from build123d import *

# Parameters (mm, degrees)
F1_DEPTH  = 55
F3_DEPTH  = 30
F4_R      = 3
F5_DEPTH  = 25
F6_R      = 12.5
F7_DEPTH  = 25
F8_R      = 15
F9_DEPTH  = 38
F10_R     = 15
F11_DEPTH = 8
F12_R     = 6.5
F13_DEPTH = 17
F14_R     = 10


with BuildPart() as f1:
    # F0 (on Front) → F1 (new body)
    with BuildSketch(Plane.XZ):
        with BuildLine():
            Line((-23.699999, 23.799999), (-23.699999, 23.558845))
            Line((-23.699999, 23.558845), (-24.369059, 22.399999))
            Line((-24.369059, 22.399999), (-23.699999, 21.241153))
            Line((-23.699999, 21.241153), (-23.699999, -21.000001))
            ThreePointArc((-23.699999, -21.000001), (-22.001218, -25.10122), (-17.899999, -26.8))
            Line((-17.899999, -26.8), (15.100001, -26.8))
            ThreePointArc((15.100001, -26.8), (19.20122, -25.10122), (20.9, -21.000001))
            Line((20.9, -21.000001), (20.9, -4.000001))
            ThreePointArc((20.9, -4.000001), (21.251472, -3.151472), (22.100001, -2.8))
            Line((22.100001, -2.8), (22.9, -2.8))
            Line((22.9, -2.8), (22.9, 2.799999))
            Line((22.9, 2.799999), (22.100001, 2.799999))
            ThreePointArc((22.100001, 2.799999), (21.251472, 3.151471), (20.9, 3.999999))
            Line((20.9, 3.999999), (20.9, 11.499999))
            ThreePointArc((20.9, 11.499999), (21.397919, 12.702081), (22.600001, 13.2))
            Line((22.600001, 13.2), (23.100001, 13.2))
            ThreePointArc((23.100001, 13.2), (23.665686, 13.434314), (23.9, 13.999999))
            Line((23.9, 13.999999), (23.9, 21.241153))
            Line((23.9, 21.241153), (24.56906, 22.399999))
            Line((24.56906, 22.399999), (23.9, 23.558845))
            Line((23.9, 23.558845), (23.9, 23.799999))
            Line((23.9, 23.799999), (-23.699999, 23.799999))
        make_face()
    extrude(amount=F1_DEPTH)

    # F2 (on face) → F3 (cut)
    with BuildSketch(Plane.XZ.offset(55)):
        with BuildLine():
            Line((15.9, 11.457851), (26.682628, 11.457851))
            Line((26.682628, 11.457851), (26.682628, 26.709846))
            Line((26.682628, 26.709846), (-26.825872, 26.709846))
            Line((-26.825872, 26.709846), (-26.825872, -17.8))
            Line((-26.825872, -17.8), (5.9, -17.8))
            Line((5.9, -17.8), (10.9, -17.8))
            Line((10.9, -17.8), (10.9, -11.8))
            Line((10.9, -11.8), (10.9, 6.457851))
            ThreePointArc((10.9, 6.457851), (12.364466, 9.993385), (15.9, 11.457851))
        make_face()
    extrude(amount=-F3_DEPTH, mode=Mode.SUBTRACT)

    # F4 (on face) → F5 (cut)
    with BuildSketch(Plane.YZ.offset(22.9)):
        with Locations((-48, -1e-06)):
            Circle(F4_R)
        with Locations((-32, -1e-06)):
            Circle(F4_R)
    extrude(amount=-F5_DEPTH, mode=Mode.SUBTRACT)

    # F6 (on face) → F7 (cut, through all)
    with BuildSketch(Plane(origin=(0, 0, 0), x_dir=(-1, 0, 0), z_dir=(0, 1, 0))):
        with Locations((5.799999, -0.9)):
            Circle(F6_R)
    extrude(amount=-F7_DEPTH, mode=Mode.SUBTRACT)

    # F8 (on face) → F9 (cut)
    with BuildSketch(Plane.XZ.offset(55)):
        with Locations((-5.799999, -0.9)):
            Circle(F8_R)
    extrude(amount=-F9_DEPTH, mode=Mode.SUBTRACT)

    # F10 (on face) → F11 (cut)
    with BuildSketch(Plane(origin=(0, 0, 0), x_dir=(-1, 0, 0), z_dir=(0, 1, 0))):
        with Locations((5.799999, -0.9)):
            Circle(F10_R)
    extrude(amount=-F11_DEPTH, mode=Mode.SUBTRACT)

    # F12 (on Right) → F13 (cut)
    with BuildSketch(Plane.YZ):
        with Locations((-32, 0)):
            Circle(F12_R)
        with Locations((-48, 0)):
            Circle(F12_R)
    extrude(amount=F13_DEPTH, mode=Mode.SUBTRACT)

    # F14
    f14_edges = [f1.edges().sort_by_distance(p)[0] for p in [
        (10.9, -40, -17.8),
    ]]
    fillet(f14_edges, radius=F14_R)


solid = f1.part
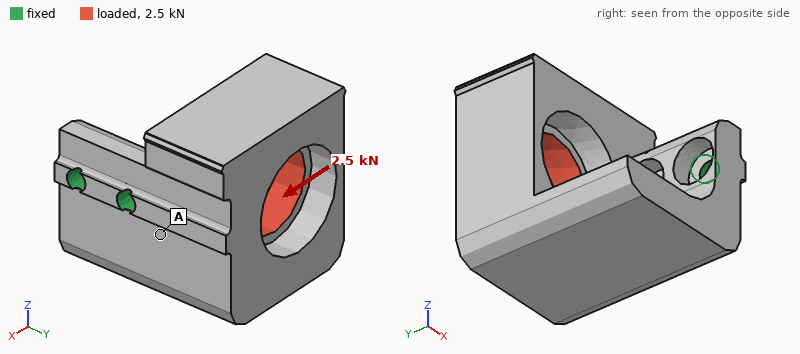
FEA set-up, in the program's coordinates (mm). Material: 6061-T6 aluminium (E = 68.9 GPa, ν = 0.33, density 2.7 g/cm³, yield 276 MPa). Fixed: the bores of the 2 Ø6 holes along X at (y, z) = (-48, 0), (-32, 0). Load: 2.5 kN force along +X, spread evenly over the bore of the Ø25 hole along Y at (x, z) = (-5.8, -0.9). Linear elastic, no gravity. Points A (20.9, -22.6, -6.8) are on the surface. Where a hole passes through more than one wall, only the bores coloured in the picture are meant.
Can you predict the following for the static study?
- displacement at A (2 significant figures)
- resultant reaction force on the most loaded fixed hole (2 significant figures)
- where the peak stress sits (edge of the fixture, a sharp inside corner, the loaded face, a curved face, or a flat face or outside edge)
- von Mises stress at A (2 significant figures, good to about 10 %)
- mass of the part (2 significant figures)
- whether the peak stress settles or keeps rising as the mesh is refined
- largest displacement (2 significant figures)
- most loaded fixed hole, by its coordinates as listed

0.031 mm
4.3 kN
edge of the fixture
17 MPa
160 g
keeps rising
0.14 mm
(-32, 0)
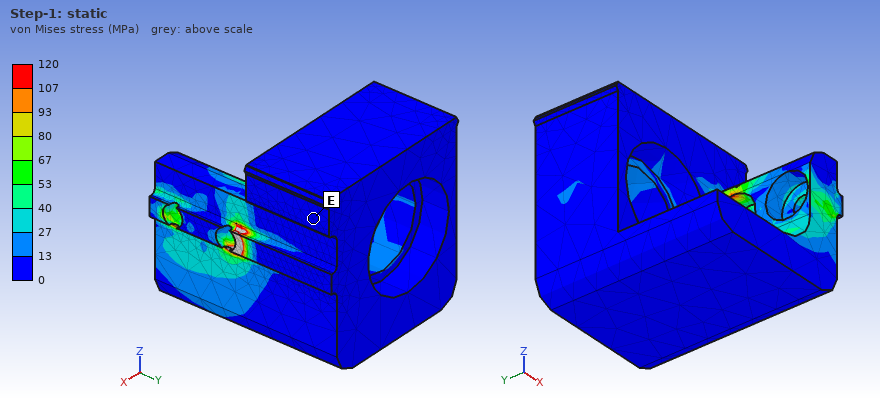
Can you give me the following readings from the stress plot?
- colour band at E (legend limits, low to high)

0 to 13 MPa
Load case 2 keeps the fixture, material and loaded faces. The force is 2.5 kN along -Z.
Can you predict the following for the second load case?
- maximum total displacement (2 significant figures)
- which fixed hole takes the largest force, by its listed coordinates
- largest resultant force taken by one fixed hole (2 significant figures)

0.41 mm
(-32, 0)
4.4 kN
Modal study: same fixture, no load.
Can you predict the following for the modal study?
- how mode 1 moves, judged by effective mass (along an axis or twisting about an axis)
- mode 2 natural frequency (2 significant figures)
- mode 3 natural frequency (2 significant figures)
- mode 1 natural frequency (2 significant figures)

along Z
2000 Hz
3900 Hz
1300 Hz
